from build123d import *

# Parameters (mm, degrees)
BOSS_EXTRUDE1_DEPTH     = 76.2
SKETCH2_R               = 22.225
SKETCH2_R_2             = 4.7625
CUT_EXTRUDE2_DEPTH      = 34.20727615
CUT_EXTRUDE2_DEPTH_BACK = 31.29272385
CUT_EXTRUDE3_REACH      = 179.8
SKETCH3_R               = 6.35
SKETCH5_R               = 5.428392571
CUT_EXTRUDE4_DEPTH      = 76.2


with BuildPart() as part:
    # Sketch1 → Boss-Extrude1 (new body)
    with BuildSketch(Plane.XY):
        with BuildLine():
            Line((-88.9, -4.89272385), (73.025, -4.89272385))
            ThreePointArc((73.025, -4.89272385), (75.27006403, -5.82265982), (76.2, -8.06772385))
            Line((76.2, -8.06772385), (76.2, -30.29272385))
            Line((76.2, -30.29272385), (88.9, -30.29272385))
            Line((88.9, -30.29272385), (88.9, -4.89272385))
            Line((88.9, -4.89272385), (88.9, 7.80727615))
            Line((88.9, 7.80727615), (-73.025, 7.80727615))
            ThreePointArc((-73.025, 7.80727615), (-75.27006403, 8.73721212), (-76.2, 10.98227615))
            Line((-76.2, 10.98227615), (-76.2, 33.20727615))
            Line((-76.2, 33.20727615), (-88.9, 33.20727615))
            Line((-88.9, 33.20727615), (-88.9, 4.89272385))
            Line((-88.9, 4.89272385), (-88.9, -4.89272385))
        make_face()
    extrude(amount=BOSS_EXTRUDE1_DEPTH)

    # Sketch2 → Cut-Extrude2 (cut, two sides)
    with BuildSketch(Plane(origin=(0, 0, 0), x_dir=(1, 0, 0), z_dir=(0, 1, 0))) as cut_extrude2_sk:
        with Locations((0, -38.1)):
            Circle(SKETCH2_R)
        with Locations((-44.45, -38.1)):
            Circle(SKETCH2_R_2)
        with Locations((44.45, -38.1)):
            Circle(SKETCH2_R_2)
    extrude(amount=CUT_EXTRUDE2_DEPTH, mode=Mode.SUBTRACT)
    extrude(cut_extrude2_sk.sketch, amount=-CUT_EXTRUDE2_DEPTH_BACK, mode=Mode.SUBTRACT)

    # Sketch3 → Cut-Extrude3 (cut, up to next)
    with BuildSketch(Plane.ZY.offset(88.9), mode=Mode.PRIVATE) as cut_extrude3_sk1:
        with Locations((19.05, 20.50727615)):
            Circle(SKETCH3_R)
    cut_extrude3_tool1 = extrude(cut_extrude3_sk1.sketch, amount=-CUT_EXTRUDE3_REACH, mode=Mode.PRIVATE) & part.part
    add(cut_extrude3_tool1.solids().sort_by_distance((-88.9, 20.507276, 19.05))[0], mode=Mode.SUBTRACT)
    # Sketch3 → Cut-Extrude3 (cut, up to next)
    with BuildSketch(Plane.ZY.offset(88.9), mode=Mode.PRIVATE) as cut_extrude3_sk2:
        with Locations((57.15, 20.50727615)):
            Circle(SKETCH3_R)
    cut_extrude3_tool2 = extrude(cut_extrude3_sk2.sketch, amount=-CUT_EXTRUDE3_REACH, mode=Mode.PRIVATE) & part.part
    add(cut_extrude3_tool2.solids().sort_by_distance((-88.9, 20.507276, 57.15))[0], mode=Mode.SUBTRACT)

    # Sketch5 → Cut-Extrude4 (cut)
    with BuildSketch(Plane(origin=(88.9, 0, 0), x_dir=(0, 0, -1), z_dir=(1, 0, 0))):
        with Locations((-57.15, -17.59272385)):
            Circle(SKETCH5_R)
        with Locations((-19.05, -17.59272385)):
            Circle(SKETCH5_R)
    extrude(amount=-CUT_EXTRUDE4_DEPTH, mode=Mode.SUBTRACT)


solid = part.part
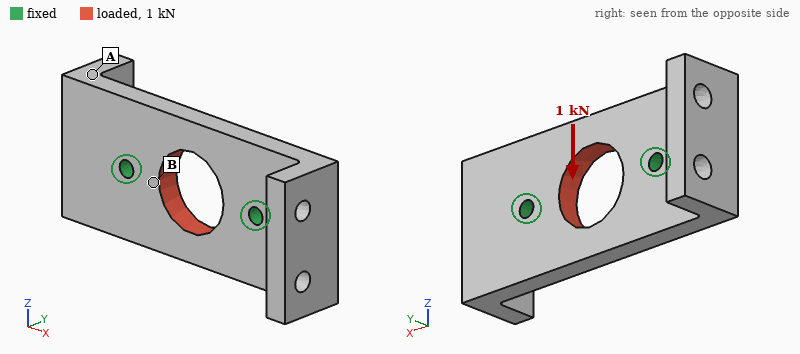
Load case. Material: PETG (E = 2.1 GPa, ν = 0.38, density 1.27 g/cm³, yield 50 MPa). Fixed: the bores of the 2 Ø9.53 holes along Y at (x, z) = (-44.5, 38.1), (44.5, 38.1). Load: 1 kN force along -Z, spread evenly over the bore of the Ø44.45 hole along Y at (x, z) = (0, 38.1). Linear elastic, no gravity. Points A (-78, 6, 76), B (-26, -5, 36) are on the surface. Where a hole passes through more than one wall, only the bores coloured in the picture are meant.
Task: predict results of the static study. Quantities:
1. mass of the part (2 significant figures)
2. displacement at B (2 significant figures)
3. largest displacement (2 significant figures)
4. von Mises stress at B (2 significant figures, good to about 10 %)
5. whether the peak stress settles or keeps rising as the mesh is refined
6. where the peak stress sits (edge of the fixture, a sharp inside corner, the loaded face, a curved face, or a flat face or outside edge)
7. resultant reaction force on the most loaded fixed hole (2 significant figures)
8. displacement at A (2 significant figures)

250 g
23 µm
46 µm
1.2 MPa
keeps rising
edge of the fixture
500 N
17 µm
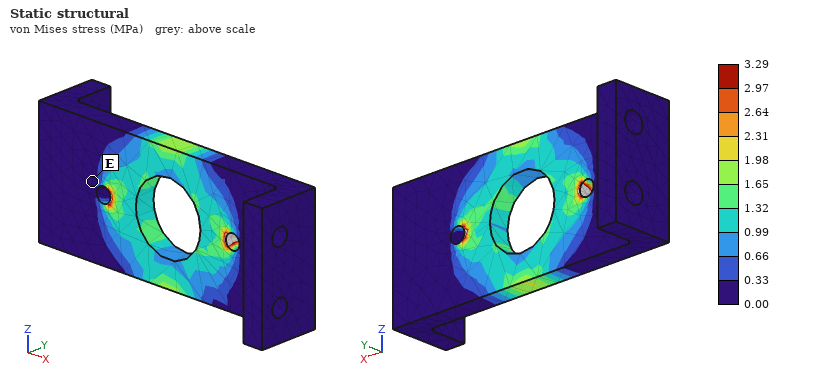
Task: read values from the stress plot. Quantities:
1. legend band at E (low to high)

0.00 to 0.33 MPa
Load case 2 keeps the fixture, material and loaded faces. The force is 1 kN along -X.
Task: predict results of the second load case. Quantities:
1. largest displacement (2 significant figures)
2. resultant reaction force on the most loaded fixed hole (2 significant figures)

22 µm
500 N
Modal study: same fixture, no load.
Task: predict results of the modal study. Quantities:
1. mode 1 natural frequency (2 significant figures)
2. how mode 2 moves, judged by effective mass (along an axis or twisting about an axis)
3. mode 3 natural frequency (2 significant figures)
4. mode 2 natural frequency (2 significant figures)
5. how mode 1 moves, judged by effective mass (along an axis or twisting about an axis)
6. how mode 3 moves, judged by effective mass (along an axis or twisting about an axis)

630 Hz
twisting about Z
740 Hz
660 Hz
along Y
twisting about X
